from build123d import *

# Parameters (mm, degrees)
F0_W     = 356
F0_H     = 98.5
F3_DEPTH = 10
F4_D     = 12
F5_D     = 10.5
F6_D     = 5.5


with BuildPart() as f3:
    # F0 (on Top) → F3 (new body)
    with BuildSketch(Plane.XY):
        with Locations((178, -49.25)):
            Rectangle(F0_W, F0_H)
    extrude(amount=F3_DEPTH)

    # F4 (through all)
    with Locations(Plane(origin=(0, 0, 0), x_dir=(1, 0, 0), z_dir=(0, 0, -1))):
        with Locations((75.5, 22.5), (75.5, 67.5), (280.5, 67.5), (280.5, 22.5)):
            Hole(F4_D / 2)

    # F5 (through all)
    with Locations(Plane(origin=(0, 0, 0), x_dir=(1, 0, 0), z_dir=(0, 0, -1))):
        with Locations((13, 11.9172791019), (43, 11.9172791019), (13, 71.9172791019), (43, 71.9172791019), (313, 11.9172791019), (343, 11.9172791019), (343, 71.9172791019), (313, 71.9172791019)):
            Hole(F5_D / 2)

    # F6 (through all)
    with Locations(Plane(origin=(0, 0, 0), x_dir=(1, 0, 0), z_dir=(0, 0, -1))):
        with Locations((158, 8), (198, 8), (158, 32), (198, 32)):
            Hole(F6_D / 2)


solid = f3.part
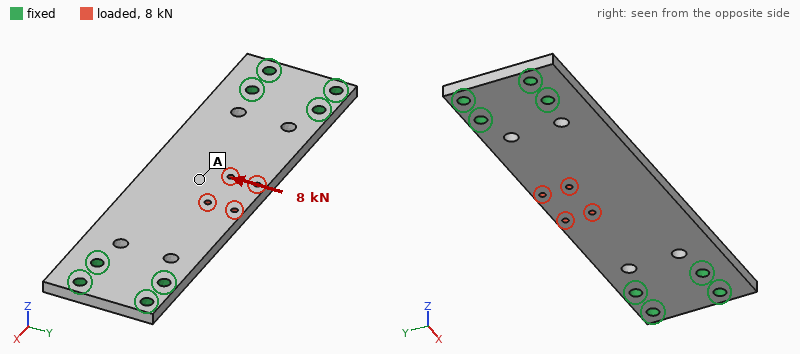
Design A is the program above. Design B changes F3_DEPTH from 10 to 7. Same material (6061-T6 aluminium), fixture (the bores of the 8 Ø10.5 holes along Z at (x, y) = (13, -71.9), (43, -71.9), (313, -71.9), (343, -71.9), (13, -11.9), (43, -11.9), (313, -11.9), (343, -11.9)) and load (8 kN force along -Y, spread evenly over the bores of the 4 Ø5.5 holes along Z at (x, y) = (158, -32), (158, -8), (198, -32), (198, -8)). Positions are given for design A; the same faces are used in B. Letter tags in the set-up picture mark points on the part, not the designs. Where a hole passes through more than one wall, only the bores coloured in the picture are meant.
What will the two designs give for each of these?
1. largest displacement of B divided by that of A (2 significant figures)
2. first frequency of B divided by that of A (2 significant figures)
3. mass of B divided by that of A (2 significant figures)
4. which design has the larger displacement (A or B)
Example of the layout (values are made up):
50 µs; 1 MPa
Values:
1.4; 0.71; 0.70; B
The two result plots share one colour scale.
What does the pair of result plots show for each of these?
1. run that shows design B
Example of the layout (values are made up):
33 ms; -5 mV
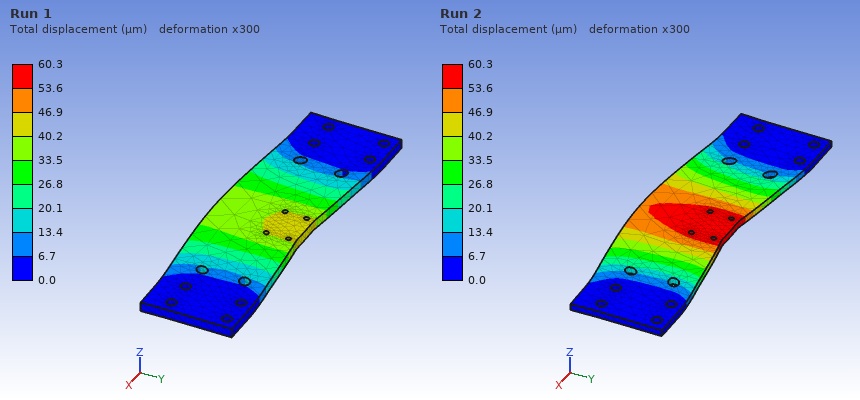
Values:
Run 2
